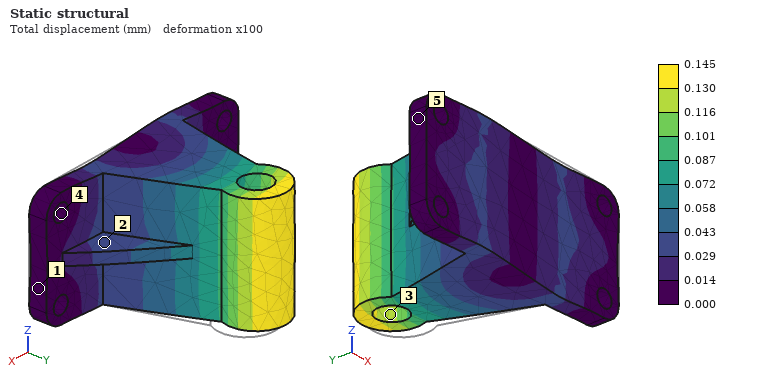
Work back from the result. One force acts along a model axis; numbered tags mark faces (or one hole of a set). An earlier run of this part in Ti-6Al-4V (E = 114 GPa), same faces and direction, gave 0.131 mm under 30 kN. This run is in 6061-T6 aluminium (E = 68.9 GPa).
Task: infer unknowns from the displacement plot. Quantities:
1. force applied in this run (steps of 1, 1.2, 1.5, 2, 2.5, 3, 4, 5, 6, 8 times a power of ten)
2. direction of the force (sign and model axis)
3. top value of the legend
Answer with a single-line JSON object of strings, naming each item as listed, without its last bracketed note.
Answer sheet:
{"force applied in this run": "20 kN", "direction of the force": "-X", "top value of the legend": "0.145 mm"}
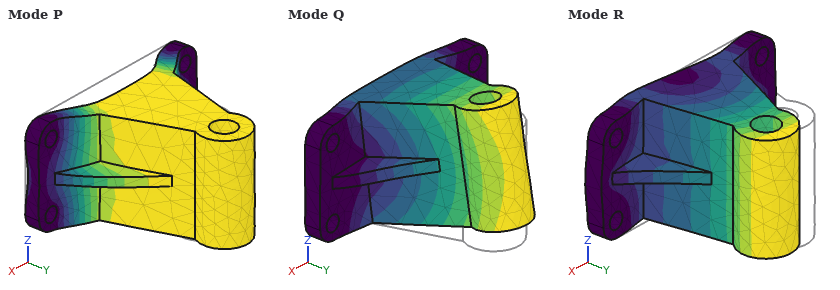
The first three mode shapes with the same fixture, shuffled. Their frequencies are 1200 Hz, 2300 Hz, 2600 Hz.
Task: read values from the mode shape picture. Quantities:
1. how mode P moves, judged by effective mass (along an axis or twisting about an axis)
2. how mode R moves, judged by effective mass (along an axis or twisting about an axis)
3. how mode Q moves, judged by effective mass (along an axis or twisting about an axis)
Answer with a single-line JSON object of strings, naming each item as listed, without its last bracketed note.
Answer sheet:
{"how mode P moves, judged by effective mass": "along Y", "how mode R moves, judged by effective mass": "along X", "how mode Q moves, judged by effective mass": "along Z"}
